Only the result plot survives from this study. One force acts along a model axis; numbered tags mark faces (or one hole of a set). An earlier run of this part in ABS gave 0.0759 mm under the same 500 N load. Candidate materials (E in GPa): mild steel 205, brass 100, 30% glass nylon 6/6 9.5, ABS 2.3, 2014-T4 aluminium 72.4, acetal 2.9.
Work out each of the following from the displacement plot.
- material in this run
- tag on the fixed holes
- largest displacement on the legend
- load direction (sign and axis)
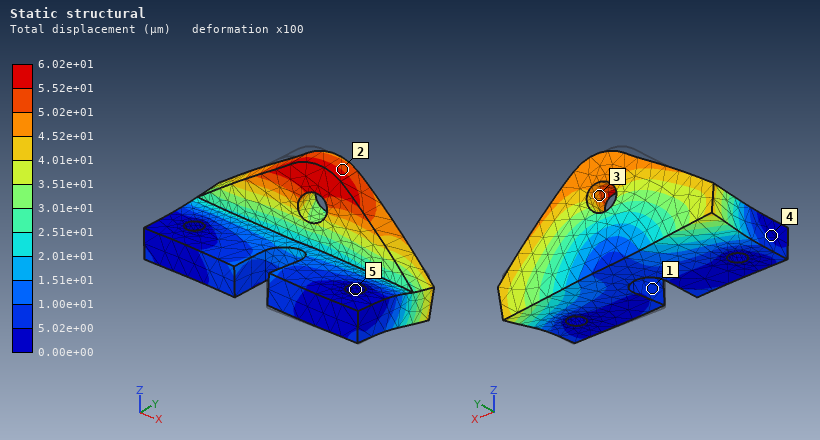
acetal
5
6.02e+01 µm
+X
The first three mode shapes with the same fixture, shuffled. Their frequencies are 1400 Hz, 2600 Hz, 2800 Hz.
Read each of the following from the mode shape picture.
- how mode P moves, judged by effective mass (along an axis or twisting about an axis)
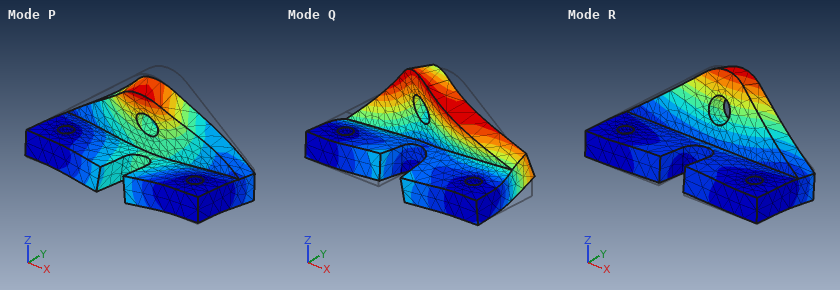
along Z
